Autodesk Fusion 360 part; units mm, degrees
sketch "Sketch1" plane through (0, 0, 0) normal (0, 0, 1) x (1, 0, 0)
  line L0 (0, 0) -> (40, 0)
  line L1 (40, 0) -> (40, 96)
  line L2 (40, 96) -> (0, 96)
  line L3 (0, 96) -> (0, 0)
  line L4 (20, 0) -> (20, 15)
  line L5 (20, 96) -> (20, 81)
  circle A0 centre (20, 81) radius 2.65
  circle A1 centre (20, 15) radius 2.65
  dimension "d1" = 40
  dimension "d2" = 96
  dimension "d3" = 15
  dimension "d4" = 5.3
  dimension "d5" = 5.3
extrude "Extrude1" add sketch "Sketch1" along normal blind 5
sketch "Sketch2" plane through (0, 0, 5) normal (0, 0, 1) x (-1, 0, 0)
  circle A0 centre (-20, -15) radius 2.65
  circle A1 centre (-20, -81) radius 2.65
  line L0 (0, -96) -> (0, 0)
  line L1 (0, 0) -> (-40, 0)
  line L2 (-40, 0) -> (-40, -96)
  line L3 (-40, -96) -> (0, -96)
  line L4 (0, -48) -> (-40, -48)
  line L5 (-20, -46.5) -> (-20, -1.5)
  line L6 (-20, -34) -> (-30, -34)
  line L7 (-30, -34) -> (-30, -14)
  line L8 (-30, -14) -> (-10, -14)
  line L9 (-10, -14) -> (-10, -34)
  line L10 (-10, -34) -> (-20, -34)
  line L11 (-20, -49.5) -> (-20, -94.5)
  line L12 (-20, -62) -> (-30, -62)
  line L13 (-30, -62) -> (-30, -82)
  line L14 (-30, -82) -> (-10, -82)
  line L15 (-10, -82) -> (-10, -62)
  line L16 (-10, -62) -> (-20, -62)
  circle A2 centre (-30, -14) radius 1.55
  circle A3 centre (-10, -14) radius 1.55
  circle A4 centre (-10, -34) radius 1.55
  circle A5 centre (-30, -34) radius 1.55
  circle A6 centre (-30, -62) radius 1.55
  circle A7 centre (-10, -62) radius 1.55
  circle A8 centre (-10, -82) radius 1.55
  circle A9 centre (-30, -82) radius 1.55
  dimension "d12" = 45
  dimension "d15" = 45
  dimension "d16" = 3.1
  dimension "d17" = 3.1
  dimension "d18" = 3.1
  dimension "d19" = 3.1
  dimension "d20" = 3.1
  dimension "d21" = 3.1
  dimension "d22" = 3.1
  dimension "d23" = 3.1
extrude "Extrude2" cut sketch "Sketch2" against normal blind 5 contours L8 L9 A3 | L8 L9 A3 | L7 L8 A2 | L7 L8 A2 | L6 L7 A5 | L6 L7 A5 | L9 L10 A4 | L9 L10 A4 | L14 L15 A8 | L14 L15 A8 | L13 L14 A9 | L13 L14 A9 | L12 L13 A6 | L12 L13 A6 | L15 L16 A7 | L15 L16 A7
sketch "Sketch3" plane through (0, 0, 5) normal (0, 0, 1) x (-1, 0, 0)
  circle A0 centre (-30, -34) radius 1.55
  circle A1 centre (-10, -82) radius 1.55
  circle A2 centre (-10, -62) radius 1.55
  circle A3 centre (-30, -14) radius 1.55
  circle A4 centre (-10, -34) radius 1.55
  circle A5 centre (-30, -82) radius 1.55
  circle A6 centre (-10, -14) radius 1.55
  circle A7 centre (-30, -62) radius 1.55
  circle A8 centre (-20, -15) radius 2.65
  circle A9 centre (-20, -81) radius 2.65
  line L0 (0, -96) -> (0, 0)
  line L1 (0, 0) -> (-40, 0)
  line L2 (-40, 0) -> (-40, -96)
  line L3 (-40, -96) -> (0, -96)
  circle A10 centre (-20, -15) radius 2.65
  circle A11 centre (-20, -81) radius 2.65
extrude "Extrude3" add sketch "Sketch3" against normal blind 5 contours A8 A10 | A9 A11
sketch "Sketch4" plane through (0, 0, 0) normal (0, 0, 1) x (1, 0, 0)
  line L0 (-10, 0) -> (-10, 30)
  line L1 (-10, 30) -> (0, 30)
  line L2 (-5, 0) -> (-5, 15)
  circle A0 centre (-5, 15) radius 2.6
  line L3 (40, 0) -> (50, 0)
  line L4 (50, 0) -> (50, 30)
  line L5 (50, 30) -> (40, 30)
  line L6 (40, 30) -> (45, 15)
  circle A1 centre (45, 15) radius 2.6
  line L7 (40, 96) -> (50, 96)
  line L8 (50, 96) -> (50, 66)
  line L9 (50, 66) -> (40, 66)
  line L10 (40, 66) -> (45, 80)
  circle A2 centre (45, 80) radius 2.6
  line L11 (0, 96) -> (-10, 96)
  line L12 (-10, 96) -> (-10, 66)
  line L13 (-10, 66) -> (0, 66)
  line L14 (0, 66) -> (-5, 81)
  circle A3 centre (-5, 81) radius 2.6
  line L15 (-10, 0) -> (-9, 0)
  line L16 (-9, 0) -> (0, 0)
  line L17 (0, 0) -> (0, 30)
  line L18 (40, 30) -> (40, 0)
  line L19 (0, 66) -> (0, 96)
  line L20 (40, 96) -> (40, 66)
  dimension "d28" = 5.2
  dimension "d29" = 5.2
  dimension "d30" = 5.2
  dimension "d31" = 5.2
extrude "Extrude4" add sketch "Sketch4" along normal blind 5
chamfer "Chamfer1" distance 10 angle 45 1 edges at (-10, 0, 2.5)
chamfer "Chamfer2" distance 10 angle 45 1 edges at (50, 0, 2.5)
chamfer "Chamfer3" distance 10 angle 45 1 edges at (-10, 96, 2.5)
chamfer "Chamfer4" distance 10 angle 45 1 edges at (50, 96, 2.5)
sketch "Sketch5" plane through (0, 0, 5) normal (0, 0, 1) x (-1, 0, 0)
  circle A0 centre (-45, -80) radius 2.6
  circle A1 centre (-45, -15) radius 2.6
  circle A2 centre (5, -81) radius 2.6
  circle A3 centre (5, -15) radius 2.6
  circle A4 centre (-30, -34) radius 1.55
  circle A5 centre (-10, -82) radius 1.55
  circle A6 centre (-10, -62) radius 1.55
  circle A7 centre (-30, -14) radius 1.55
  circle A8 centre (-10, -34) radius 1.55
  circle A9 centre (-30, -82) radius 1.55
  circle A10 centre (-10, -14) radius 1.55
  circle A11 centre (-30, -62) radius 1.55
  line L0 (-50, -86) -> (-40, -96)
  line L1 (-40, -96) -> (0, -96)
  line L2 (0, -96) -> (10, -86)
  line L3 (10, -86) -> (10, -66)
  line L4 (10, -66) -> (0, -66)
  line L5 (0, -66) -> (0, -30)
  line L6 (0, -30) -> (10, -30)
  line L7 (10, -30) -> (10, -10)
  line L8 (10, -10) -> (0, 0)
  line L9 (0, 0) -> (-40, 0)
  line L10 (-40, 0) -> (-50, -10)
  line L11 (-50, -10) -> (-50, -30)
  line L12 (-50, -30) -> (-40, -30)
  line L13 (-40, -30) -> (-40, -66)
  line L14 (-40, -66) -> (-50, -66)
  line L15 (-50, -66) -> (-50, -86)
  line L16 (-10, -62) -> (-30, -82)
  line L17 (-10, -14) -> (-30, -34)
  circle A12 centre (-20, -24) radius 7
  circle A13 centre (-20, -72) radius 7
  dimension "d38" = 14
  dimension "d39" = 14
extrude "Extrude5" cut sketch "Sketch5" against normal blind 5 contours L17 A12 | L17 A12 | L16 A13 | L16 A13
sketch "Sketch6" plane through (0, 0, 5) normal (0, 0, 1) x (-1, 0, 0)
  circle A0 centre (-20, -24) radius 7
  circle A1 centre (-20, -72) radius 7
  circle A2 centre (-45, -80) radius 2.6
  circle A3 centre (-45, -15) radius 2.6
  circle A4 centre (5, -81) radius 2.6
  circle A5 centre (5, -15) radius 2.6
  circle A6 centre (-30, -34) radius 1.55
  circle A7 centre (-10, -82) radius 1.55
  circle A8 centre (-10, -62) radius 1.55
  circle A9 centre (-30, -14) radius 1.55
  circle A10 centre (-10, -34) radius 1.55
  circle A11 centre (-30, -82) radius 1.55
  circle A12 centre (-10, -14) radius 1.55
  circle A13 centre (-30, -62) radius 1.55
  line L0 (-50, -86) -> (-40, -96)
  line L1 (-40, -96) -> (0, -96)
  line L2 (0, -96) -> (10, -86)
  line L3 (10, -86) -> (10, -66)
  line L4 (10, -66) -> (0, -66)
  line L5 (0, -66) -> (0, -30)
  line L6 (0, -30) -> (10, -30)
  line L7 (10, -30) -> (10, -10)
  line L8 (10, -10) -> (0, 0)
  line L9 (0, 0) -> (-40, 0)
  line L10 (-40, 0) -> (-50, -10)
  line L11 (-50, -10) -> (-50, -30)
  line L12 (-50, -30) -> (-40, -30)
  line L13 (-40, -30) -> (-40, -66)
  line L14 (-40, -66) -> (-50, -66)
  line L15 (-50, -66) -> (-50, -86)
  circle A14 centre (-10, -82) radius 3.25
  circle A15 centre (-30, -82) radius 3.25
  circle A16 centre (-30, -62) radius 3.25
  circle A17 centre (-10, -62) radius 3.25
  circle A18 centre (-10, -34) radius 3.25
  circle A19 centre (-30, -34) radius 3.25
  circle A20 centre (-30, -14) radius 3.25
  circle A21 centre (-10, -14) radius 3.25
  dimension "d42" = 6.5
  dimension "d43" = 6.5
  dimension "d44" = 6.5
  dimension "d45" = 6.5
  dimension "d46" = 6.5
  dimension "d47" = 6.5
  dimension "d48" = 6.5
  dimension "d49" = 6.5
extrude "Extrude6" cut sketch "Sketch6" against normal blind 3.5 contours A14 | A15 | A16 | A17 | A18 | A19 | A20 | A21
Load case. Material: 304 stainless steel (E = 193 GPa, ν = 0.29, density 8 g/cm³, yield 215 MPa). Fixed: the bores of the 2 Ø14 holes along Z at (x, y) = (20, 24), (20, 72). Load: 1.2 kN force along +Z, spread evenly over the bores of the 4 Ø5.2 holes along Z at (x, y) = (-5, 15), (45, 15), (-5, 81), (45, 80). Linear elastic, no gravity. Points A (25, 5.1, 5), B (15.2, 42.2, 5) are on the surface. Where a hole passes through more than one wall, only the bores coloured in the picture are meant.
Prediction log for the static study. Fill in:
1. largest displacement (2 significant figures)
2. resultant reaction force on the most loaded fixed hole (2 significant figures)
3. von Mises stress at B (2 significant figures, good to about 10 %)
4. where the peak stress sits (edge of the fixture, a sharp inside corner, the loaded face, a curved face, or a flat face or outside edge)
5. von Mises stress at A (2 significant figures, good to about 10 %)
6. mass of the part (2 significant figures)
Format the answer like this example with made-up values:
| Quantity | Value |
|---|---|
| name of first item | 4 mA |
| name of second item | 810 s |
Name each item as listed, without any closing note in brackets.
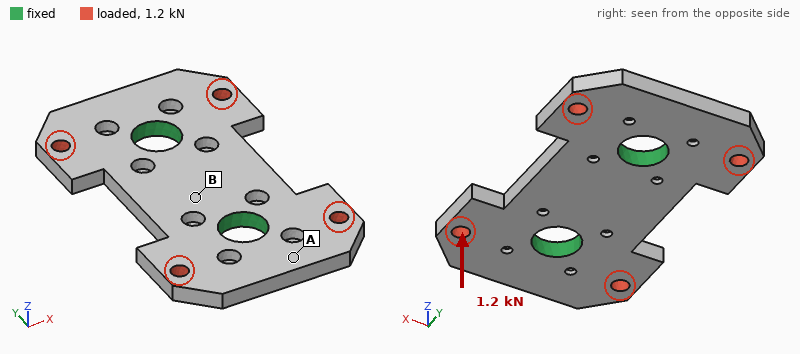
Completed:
| Quantity | Value |
|---|---|
| largest displacement | 23 µm |
| resultant reaction force on the most loaded fixed hole | 600 N |
| von Mises stress at B | 6.8 MPa |
| where the peak stress sits | a curved face |
| von Mises stress at A | 29 MPa |
| mass of the part | 170 g |
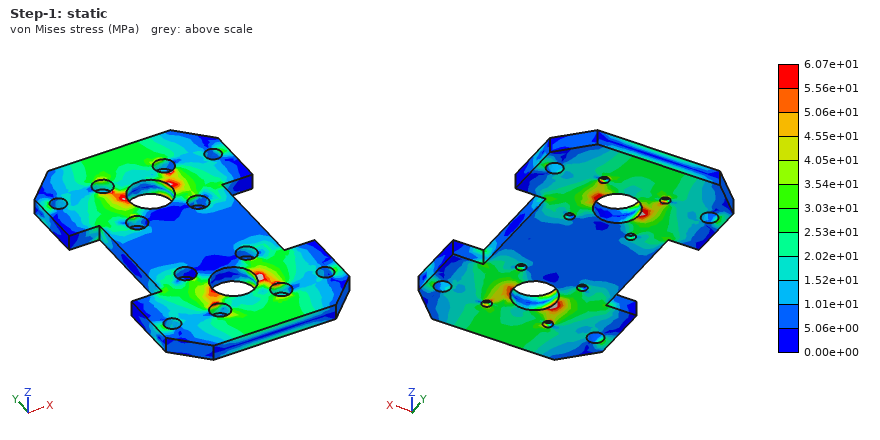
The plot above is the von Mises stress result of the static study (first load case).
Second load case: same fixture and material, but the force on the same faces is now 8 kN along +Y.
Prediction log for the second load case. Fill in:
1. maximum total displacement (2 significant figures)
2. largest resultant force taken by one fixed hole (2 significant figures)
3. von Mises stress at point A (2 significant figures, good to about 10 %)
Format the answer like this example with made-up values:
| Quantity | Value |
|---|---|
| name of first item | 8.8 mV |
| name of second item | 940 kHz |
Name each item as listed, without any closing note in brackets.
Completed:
| Quantity | Value |
|---|---|
| maximum total displacement | 7.5 µm |
| largest resultant force taken by one fixed hole | 4.0 kN |
| von Mises stress at point A | 23 MPa |
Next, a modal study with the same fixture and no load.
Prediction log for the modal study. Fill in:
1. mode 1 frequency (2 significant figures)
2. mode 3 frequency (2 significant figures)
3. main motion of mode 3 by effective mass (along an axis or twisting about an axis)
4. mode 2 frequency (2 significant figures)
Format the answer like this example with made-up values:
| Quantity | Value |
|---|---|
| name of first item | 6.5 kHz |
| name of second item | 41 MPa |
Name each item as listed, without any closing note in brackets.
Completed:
| Quantity | Value |
|---|---|
| mode 1 frequency | 6000 Hz |
| mode 3 frequency | 6500 Hz |
| main motion of mode 3 by effective mass | along Z |
| mode 2 frequency | 6100 Hz |
